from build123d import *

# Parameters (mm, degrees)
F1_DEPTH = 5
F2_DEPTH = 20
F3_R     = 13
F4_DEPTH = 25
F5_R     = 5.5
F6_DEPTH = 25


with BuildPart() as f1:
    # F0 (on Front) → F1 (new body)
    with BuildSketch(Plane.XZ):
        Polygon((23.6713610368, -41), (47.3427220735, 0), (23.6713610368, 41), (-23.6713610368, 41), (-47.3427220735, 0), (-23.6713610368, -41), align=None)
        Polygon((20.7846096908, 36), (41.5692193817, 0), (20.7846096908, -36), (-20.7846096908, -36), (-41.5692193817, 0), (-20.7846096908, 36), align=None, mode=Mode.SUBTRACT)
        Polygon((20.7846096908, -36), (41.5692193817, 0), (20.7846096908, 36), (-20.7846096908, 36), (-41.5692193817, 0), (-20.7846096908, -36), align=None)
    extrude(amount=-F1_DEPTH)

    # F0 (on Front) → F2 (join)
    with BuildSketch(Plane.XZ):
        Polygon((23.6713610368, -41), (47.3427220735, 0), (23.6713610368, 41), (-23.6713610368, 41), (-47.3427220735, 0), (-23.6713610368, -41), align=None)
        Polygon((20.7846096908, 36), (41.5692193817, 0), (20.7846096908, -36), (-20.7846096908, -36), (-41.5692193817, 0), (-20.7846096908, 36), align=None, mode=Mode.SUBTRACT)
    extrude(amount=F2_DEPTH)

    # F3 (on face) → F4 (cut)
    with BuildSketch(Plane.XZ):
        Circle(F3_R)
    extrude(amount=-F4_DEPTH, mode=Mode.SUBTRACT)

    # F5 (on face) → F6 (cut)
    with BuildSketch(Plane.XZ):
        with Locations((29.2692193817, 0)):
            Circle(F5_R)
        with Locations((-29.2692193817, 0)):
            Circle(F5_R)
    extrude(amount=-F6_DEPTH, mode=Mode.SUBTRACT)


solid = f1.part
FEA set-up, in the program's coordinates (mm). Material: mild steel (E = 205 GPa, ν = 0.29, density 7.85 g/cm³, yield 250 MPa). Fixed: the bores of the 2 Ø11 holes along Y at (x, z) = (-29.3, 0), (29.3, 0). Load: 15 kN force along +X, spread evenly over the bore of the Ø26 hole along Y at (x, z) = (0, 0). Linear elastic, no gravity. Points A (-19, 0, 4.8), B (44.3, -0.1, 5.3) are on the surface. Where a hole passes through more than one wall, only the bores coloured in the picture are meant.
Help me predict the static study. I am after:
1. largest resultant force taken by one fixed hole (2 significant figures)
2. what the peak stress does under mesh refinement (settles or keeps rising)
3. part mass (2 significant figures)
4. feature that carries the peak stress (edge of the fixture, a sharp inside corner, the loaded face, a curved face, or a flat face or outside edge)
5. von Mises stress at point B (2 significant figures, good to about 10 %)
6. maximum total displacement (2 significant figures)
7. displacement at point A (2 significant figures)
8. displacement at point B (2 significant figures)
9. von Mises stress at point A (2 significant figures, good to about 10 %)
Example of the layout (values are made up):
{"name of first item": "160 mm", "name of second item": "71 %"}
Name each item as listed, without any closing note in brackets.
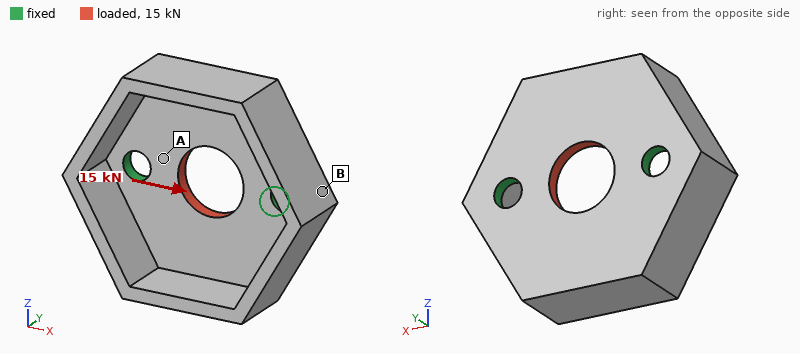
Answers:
{"largest resultant force taken by one fixed hole": "7.5 kN", "what the peak stress does under mesh refinement": "keeps rising", "part mass": "410 g", "feature that carries the peak stress": "edge of the fixture", "von Mises stress at point B": "14 MPa", "maximum total displacement": "6.8 µm", "displacement at point A": "2.1 µm", "displacement at point B": "1.1 µm", "von Mises stress at point A": "60 MPa"}
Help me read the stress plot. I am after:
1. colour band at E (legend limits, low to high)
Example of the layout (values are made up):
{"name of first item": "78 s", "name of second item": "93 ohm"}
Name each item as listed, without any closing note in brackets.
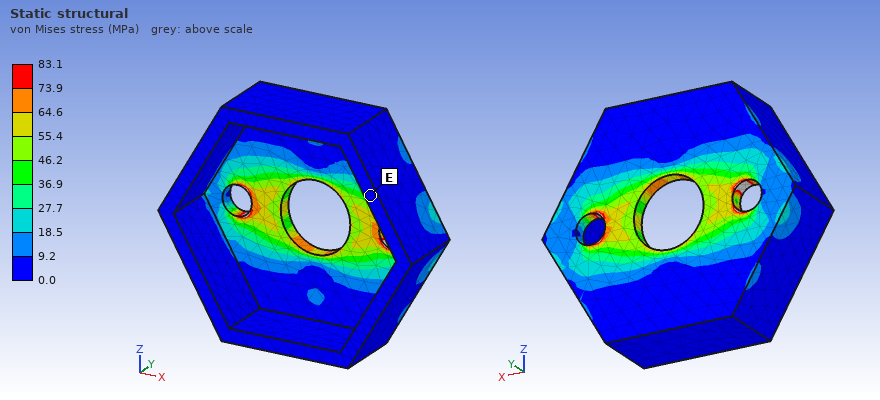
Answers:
{"colour band at E": "0.0 to 9.2 MPa"}
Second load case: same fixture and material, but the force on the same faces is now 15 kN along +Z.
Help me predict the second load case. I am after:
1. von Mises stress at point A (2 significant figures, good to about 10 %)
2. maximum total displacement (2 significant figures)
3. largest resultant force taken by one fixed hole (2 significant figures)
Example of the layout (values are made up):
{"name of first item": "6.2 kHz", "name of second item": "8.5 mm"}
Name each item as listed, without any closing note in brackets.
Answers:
{"von Mises stress at point A": "58 MPa", "maximum total displacement": "8.4 µm", "largest resultant force taken by one fixed hole": "7.5 kN"}
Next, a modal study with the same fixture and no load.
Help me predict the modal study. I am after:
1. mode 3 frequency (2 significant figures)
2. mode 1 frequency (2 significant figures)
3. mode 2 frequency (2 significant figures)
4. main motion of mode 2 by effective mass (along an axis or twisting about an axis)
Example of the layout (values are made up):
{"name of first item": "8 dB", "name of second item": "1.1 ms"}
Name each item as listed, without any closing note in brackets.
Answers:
{"mode 3 frequency": "4200 Hz", "mode 1 frequency": "2400 Hz", "mode 2 frequency": "3400 Hz", "main motion of mode 2 by effective mass": "along Y"}
